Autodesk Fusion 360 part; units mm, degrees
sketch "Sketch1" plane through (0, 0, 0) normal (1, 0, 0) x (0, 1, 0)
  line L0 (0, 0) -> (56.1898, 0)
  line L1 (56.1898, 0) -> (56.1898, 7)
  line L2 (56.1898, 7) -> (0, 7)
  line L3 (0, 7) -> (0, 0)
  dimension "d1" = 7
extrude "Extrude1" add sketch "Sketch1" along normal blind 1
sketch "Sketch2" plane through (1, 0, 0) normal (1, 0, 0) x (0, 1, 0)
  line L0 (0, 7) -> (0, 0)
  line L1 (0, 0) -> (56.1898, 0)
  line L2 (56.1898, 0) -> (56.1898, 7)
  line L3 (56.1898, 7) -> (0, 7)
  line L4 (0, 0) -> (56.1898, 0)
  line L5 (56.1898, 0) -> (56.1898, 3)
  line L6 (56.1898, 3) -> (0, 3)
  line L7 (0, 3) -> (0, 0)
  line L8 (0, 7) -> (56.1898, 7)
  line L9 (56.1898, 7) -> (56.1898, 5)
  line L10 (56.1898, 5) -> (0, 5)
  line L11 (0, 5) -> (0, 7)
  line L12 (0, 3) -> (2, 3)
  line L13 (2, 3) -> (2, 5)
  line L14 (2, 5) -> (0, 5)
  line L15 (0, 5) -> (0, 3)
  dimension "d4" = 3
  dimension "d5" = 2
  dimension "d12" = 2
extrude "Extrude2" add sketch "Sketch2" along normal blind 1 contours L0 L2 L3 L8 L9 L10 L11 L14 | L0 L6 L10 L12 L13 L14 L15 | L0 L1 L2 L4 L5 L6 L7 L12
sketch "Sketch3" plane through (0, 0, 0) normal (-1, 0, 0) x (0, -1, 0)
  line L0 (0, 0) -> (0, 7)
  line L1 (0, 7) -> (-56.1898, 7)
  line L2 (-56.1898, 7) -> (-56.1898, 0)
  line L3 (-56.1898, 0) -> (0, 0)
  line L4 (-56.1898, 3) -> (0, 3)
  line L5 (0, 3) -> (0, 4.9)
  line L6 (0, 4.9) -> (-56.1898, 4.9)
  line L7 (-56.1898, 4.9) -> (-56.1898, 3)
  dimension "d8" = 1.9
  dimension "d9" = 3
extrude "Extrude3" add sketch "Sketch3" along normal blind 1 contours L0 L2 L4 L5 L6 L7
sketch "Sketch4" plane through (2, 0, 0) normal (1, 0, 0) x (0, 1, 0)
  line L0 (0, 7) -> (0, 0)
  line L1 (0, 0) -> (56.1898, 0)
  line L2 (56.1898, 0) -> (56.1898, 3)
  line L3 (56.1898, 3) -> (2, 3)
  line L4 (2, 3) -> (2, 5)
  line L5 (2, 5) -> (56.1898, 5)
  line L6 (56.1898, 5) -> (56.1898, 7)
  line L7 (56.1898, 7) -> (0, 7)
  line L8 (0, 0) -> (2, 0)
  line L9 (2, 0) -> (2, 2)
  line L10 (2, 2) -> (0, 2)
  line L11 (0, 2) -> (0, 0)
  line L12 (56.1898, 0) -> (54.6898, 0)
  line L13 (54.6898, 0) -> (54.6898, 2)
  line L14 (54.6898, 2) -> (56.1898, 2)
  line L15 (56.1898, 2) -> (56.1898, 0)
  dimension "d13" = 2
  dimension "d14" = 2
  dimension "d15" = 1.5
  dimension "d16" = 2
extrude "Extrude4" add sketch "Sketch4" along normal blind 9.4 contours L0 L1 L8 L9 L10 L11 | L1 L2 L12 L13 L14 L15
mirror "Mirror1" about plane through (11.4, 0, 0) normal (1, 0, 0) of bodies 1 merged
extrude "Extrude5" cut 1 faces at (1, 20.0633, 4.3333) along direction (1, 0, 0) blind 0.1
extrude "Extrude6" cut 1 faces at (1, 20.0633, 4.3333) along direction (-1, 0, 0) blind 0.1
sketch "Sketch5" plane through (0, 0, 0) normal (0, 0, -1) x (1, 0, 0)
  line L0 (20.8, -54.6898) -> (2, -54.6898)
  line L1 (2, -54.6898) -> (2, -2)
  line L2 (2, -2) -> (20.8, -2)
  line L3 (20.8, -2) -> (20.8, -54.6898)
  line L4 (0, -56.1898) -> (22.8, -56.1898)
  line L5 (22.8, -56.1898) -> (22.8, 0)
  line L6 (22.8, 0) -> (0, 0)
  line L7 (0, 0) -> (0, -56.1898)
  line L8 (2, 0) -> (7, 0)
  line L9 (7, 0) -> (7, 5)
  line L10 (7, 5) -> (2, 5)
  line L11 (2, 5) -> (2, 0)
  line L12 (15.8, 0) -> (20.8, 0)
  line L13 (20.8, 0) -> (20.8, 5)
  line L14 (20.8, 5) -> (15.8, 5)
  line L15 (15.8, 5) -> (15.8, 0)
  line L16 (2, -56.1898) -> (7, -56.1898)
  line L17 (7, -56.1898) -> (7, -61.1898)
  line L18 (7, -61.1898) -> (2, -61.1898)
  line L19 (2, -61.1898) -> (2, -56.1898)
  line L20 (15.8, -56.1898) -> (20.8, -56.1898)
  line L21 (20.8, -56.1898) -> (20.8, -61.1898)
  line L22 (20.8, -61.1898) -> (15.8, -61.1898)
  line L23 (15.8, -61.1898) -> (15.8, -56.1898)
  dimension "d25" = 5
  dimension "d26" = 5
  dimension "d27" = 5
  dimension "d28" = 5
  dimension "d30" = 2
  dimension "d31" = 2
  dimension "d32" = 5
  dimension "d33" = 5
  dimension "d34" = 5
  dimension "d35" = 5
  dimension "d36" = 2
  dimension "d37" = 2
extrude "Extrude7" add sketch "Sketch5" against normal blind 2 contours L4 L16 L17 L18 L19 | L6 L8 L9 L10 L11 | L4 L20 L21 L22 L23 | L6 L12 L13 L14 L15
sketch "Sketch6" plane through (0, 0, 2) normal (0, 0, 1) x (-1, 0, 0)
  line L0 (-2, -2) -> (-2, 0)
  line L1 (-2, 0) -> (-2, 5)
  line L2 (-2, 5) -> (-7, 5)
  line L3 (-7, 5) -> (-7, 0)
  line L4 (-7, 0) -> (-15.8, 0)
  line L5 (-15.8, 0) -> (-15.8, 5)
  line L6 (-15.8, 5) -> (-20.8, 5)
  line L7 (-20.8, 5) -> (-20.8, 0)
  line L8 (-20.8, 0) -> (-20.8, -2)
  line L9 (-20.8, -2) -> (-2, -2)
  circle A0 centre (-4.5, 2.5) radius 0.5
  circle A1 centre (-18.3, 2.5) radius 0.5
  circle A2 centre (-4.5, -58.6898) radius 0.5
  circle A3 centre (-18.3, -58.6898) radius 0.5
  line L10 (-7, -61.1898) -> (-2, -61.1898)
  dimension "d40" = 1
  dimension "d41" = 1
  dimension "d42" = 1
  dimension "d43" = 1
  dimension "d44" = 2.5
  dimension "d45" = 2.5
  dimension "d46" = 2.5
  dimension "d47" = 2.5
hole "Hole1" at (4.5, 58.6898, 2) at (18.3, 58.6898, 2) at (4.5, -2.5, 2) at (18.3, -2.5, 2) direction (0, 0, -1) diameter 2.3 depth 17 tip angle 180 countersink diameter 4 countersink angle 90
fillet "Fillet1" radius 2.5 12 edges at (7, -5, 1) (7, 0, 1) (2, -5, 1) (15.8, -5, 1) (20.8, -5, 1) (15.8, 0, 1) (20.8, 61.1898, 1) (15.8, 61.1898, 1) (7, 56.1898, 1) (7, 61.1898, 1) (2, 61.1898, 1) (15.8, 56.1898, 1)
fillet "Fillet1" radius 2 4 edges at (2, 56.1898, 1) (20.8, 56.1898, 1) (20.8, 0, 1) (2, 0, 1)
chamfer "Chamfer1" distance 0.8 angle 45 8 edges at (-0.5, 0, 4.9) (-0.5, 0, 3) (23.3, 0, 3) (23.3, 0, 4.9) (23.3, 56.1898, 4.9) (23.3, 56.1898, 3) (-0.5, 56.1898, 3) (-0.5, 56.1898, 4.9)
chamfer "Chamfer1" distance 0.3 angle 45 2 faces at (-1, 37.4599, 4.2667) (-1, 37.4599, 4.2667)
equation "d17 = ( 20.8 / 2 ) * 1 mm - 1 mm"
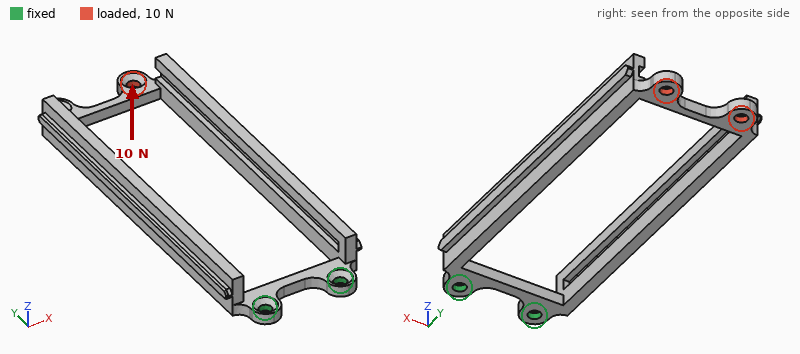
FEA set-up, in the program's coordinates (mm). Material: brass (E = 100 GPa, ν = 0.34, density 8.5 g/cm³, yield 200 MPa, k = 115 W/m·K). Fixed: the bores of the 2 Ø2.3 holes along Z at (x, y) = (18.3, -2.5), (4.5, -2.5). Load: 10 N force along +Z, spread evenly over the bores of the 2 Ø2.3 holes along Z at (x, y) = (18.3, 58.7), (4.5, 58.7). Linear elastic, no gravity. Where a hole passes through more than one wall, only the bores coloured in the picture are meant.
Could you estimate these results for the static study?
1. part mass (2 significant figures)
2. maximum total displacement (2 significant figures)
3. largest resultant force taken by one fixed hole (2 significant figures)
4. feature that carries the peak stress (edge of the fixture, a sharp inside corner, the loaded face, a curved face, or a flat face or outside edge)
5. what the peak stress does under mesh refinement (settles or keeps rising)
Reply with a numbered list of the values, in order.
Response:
1. 16 g
2. 0.46 mm
3. 5.3 N
4. edge of the fixture
5. keeps rising
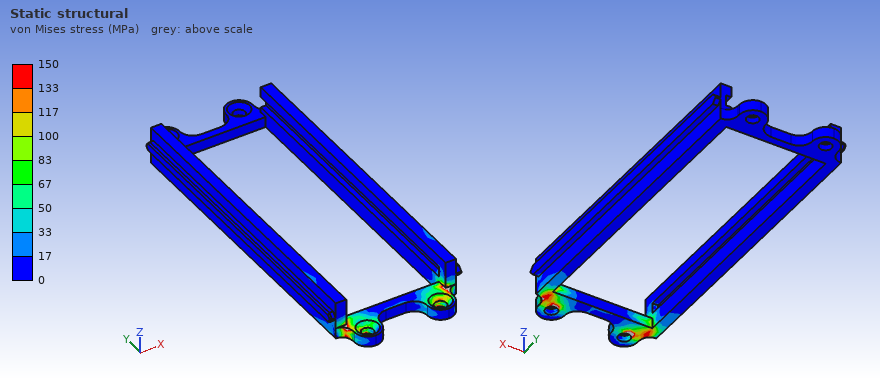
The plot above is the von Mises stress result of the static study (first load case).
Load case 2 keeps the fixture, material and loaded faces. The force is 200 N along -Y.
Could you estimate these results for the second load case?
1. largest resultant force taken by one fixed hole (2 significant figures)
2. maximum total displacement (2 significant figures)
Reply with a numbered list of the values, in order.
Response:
1. 110 N
2. 0.17 mm
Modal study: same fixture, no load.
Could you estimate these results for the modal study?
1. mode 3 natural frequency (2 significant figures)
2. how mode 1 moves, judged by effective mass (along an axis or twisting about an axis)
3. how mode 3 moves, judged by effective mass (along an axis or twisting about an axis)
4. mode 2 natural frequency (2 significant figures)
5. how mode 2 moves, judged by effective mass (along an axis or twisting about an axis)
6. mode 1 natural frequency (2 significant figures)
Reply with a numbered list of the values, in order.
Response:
1. 780 Hz
2. along Z
3. twisting about Y
4. 440 Hz
5. along X
6. 350 Hz
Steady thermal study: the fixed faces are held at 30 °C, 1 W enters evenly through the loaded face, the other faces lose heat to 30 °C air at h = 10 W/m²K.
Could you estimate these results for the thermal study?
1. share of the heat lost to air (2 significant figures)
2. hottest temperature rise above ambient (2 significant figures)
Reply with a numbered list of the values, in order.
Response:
1. 27 %
2. 21 K
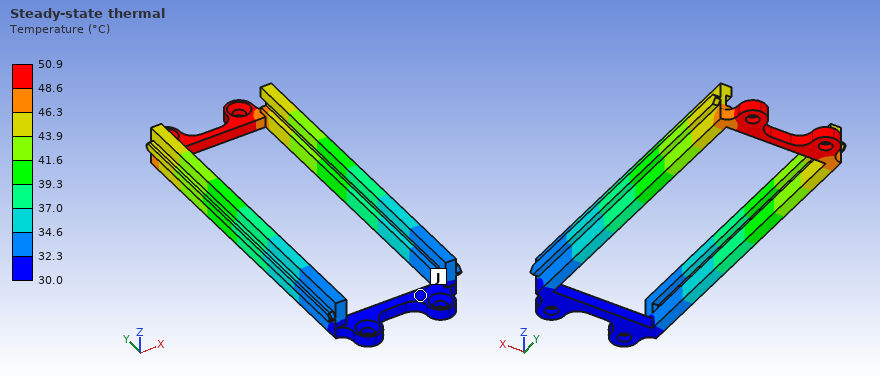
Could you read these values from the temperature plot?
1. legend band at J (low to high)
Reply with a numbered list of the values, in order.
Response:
1. 30.0 to 32.3 °C
